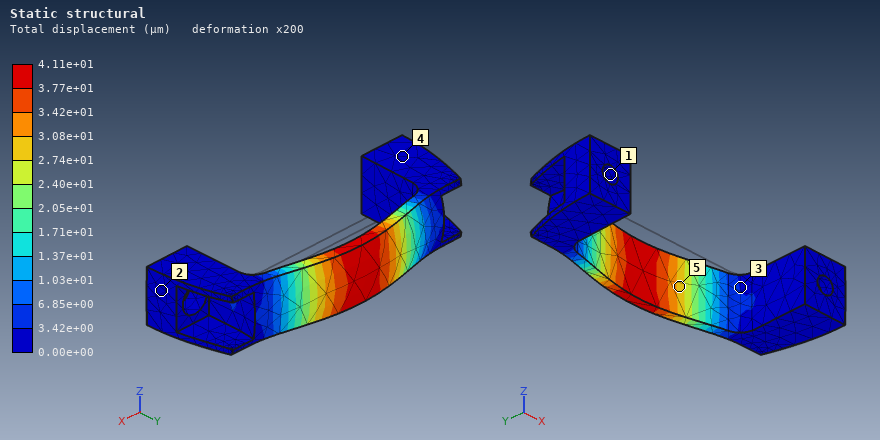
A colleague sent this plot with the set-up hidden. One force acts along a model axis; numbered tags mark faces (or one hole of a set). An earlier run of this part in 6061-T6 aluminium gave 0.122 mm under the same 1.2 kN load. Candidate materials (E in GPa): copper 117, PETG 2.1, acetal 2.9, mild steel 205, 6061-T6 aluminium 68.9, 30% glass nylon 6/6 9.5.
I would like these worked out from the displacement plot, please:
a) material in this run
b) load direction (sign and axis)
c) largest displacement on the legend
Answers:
mild steel
+Y
4.11e+01 µm
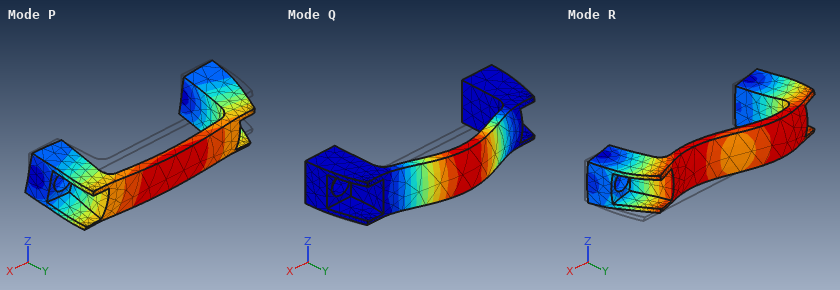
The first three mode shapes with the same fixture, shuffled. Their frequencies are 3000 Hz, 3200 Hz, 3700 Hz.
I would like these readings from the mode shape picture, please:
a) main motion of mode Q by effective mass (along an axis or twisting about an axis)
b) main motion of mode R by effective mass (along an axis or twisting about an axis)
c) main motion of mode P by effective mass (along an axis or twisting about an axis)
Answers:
along Y
along X
along Z
